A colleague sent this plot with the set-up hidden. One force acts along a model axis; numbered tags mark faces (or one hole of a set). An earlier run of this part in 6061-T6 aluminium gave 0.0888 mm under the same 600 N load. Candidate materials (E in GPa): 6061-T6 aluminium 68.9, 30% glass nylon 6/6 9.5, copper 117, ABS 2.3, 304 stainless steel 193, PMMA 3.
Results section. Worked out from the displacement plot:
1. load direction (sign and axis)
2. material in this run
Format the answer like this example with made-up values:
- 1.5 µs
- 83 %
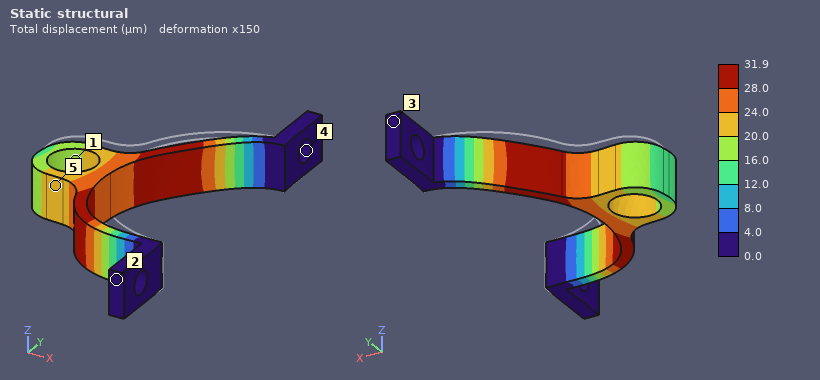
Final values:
- -Y
- 304 stainless steel
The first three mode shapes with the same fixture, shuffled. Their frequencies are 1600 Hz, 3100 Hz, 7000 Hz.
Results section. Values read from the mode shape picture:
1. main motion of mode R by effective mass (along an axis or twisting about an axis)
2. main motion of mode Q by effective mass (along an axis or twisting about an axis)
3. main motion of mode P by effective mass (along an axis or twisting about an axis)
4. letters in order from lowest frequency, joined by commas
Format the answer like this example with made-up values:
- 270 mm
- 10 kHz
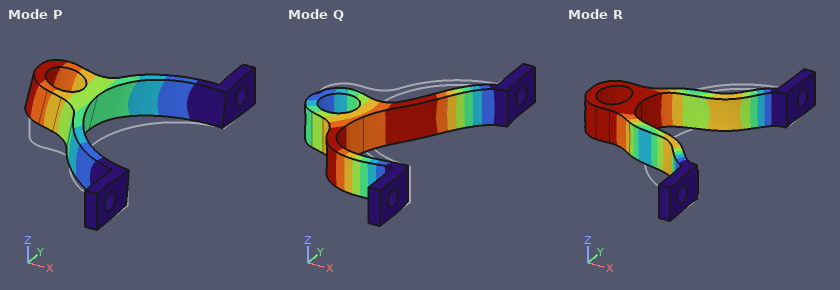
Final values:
- along X
- along Y
- along Z
- P, Q, R
